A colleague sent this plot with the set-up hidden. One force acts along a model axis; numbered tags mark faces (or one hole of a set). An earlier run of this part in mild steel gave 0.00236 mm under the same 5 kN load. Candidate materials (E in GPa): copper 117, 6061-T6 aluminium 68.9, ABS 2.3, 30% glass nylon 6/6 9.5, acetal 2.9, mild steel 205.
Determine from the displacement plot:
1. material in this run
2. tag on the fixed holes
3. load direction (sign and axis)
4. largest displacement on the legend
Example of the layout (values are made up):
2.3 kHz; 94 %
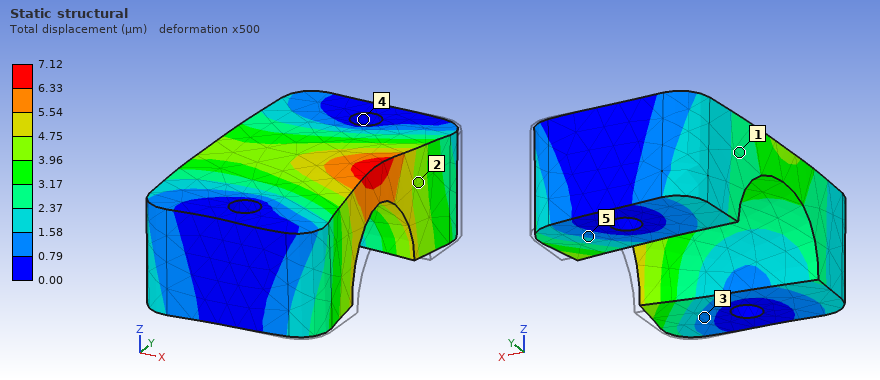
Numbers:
6061-T6 aluminium; 4; -X; 7.12 µm
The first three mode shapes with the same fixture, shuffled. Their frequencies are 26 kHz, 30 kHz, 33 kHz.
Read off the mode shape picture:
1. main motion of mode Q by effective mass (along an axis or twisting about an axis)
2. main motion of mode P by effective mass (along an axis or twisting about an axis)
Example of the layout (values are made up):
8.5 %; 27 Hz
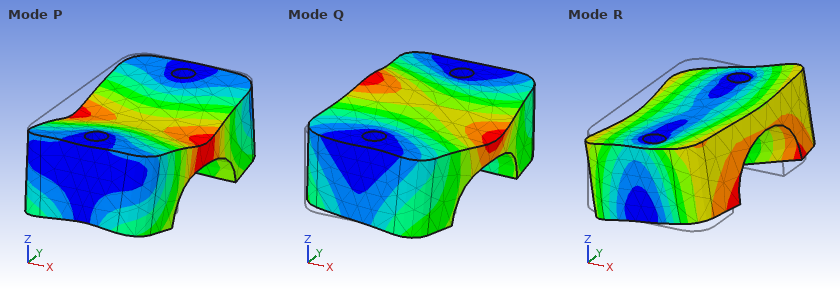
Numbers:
along X; along Z
